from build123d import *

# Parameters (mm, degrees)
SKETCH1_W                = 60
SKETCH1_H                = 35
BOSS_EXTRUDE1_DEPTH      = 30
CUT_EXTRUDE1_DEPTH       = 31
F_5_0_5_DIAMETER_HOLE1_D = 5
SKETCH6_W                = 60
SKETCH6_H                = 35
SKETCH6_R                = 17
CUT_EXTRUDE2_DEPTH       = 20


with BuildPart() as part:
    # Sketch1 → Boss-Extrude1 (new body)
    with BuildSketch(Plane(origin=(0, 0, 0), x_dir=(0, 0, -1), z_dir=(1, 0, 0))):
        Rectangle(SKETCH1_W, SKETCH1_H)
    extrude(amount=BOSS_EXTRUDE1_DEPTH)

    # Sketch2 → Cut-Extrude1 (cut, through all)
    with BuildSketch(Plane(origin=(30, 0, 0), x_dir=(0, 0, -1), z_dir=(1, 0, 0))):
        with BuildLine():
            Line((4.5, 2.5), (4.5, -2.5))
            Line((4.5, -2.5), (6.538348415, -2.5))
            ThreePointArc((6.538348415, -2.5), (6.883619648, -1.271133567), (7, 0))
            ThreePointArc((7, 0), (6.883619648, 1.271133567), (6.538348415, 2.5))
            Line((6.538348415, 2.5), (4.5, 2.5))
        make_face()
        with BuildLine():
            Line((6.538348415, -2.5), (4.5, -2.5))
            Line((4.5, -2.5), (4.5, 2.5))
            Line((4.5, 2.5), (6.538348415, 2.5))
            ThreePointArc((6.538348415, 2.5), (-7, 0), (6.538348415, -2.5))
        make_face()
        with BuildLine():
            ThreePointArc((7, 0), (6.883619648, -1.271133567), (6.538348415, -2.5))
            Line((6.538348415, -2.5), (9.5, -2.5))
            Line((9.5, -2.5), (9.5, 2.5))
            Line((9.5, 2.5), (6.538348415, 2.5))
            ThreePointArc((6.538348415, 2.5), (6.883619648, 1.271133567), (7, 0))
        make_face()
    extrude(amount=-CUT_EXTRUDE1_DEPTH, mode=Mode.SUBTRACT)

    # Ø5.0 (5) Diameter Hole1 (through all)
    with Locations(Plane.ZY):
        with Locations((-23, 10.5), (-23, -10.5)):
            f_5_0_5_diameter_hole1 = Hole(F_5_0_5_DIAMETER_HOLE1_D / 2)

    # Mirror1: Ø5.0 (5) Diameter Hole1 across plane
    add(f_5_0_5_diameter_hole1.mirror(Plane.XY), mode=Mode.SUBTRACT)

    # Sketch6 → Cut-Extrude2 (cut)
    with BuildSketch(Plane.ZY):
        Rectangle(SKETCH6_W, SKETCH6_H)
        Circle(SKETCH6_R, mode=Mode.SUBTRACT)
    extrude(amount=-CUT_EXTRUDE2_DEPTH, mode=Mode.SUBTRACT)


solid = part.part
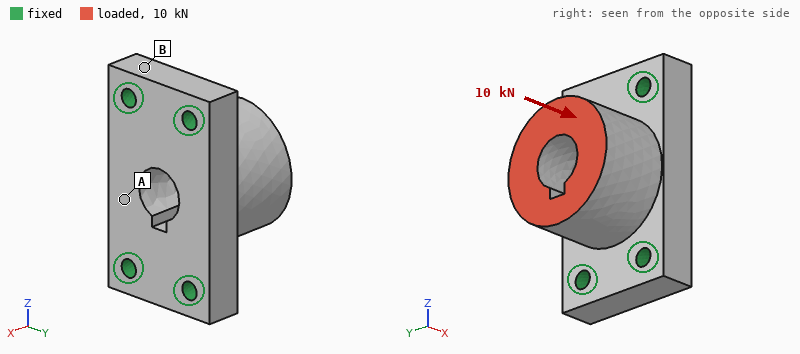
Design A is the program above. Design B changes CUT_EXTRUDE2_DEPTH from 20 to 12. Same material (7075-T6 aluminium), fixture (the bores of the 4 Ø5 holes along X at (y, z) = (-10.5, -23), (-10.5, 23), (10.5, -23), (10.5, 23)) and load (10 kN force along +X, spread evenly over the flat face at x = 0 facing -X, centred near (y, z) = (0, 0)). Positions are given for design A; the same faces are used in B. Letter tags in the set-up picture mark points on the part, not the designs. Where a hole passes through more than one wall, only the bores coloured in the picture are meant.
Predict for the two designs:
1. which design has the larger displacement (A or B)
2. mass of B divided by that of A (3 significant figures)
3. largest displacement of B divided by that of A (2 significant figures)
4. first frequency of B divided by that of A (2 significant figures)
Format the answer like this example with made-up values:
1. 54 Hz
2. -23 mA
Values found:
1. A
2. 1.27
3. 0.57
4. 1.8
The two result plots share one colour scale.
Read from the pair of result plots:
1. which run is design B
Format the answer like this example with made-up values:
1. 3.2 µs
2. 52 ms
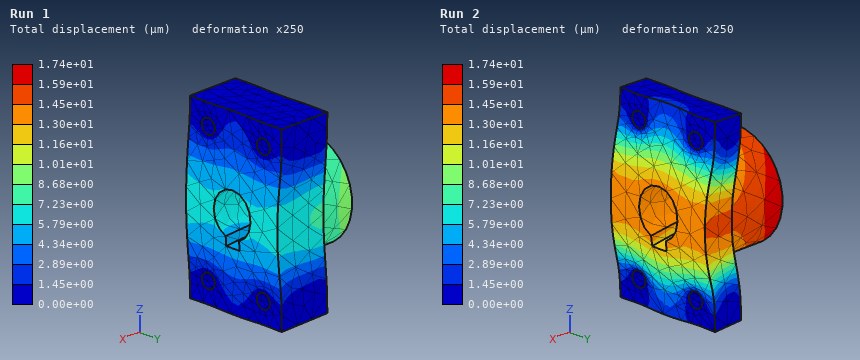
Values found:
1. Run 1
